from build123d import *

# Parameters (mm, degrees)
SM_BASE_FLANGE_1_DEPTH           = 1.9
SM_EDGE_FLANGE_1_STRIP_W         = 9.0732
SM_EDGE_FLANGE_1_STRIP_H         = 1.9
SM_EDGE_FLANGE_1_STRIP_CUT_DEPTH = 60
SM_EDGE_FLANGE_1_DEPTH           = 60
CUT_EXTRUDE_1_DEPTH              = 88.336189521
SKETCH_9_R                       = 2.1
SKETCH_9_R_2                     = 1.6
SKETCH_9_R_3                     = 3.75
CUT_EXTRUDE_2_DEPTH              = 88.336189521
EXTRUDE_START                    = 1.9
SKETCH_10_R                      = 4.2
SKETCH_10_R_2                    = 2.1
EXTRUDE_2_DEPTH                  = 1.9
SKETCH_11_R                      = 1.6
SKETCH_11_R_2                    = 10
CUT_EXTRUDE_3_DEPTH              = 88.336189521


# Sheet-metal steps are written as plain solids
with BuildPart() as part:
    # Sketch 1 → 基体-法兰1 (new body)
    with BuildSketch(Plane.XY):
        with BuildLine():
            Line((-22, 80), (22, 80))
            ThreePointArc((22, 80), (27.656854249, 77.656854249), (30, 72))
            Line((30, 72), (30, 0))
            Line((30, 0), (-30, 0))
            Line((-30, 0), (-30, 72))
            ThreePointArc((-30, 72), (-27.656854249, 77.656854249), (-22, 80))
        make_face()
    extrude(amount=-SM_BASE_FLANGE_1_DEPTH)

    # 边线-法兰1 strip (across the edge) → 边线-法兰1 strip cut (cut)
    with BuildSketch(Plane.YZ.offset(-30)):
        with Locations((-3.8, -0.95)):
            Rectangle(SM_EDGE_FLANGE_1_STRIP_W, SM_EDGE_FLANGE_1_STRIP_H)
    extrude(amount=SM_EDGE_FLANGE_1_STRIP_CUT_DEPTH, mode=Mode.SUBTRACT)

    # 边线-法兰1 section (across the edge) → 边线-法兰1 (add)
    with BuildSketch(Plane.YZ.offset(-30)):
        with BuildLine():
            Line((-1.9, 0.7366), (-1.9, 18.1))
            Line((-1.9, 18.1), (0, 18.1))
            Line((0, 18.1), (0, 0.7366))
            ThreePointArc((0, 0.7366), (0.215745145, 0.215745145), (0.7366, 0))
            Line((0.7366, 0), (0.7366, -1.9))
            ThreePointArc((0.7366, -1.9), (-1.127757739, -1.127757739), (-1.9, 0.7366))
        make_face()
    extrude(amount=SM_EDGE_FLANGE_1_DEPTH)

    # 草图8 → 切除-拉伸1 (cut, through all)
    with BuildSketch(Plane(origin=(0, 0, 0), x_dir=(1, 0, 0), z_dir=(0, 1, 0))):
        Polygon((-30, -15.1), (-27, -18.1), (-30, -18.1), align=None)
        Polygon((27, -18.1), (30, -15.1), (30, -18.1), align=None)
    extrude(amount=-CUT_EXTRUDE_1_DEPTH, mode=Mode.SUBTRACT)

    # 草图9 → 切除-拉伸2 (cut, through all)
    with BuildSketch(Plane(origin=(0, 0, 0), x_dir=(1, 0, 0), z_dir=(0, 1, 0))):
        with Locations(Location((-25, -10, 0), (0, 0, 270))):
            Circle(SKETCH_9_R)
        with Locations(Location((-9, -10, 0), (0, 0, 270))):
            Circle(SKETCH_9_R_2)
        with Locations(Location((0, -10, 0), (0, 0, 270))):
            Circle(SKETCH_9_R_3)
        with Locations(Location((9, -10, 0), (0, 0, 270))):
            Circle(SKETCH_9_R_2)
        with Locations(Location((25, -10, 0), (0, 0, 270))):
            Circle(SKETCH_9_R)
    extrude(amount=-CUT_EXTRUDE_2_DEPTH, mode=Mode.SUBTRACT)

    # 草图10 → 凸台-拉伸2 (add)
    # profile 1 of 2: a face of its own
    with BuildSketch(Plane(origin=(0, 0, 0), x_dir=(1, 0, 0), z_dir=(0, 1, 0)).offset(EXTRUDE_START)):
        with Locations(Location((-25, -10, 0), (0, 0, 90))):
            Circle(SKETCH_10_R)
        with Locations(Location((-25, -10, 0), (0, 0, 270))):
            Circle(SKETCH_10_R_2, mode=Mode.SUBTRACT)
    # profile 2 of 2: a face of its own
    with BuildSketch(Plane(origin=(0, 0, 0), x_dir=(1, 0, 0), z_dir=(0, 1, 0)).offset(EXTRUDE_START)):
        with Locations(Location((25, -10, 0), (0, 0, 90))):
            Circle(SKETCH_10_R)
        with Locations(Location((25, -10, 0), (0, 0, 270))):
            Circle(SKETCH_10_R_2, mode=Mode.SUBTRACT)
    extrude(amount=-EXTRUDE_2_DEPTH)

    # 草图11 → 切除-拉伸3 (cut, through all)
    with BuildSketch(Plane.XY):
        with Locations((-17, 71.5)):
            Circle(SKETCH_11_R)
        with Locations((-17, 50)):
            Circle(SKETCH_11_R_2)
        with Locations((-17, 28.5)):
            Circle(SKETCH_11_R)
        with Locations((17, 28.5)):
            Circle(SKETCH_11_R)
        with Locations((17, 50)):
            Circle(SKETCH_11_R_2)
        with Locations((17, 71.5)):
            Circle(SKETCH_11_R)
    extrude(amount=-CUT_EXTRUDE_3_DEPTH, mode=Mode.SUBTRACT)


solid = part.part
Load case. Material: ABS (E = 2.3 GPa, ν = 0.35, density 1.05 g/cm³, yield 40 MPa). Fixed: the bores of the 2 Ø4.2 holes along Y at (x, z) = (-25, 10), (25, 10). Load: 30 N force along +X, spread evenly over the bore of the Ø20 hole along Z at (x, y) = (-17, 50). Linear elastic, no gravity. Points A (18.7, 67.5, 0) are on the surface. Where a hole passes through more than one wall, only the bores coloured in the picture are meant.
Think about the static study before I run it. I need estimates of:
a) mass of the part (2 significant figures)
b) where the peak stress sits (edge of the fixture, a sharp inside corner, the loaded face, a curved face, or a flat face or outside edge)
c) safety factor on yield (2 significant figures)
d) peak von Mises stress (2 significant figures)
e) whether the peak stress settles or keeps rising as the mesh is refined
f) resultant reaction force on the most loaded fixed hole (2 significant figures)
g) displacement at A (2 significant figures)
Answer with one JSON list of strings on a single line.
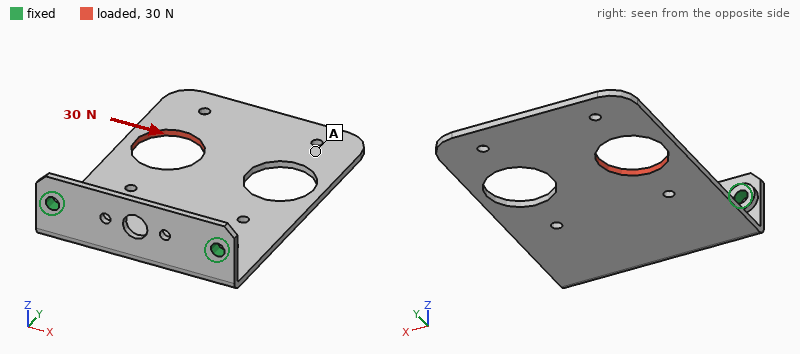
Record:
["10 g", "a flat face or outside edge", "1.9", "21 MPa", "settles", "35 N", "0.85 mm"]
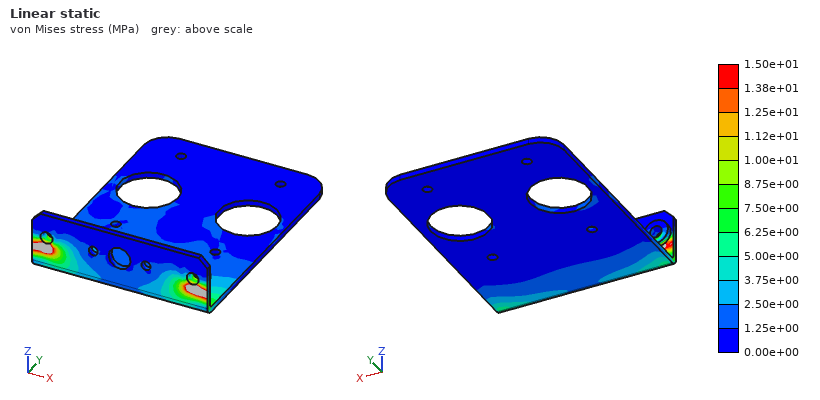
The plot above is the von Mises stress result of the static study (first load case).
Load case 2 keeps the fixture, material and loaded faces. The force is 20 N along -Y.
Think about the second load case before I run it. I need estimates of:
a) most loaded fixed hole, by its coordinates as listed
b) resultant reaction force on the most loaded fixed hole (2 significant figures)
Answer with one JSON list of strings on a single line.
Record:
["(-25, 10)", "17 N"]
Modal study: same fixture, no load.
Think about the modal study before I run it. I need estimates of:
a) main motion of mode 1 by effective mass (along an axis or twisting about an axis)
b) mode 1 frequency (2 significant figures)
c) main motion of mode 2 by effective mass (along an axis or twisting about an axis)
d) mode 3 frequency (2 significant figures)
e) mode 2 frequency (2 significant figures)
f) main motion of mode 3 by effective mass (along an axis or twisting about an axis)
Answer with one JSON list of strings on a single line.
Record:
["along Z", "62 Hz", "twisting about Y", "330 Hz", "210 Hz", "along Z"]
